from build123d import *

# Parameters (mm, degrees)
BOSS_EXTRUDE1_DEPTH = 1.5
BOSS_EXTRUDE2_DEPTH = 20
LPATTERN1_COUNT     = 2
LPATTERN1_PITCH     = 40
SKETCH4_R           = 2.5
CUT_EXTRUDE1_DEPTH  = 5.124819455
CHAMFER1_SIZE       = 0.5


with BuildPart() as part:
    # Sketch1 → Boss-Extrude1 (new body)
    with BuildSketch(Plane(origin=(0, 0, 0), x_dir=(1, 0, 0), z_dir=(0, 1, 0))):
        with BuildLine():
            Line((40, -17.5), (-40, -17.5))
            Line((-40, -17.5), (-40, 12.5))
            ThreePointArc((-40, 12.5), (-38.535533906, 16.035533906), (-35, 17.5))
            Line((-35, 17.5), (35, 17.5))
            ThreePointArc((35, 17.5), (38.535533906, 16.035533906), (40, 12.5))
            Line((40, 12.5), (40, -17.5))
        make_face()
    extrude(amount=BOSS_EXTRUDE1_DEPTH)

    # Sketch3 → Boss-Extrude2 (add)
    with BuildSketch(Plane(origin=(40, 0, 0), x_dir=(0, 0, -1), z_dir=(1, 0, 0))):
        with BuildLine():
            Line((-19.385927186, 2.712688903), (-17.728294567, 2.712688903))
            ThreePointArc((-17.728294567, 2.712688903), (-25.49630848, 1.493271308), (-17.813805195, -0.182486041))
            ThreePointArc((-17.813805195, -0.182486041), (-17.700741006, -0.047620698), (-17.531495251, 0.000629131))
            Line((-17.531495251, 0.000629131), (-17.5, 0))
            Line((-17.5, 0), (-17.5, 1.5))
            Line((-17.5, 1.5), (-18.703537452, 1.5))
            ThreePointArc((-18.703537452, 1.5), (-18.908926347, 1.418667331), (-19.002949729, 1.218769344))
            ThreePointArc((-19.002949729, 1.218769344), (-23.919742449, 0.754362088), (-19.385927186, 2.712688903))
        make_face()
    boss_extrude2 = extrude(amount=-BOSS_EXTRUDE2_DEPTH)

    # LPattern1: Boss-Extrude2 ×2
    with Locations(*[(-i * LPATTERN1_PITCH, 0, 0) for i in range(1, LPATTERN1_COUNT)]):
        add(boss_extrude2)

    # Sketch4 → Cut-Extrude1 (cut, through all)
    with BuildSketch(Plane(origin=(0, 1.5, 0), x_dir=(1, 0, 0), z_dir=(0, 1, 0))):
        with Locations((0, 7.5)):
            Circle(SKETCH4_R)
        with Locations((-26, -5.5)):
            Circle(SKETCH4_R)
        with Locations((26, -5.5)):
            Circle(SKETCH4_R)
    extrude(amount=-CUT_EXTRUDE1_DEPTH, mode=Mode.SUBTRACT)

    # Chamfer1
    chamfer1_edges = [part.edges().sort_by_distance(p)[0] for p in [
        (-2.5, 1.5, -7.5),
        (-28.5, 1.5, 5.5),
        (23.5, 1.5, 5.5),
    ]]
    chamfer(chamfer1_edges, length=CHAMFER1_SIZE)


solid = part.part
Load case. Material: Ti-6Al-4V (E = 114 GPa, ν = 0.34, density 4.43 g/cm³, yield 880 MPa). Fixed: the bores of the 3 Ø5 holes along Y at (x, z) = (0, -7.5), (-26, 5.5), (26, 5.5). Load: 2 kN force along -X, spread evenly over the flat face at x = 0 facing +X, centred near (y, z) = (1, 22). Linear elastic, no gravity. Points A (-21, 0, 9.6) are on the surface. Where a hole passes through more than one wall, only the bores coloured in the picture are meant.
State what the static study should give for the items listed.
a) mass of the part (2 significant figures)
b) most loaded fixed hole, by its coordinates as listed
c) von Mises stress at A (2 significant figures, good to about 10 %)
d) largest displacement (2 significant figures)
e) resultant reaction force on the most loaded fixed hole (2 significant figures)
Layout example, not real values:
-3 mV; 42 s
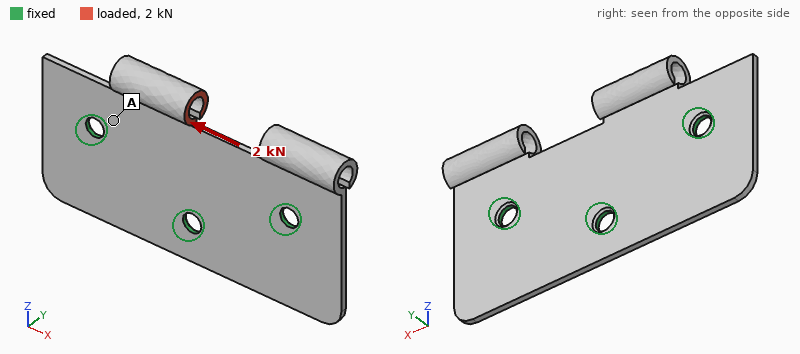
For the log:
23 g; (-26, 5.5); 110 MPa; 0.49 mm; 1.5 kN
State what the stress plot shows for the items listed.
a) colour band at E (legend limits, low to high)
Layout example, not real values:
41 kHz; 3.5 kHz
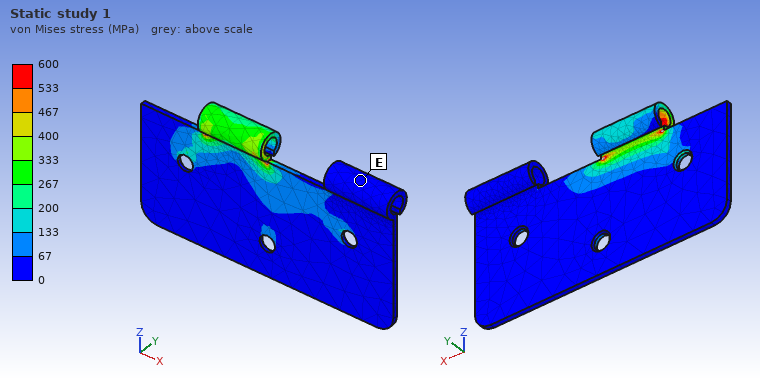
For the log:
0 to 67 MPa
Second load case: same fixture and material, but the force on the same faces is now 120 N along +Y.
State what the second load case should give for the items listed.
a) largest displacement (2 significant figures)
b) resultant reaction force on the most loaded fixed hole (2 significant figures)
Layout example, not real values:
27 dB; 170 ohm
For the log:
0.48 mm; 55 N
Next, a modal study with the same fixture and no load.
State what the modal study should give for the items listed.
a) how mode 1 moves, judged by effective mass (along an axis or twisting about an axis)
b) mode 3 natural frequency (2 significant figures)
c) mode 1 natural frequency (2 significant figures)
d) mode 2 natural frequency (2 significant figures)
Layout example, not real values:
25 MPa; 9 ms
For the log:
along Y; 3000 Hz; 2000 Hz; 2200 Hz
